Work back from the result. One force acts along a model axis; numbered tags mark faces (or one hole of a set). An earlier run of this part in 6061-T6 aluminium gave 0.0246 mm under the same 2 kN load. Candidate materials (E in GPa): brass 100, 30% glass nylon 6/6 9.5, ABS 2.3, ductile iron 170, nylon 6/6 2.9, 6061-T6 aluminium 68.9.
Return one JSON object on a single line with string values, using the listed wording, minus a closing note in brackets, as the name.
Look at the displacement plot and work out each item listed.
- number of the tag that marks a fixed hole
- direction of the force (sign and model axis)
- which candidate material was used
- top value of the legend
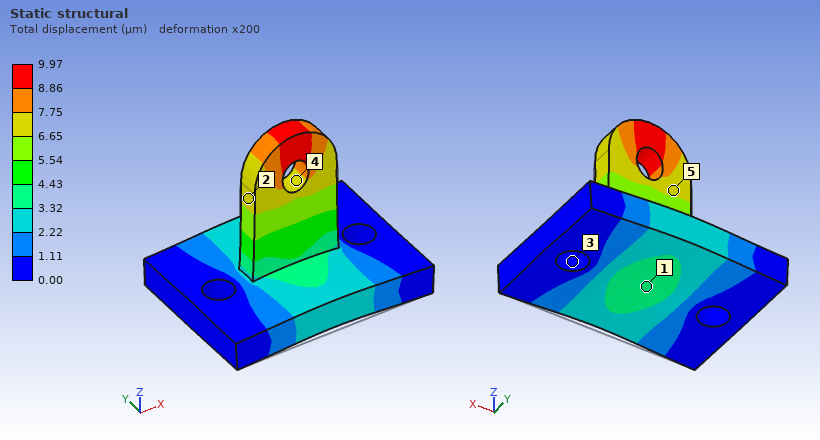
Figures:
{"number of the tag that marks a fixed hole": "3", "direction of the force": "+Z", "which candidate material was used": "ductile iron", "top value of the legend": "9.97 µm"}
